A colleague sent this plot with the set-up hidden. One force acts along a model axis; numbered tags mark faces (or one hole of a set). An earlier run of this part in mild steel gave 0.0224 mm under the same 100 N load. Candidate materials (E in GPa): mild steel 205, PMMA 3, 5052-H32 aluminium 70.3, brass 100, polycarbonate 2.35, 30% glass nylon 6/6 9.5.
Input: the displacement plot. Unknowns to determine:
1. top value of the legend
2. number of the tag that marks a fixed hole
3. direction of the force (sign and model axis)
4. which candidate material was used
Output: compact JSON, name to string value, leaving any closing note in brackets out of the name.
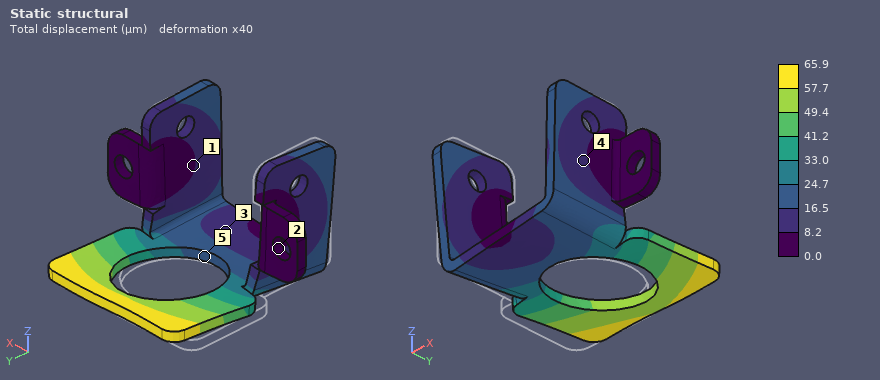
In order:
{"top value of the legend": "65.9 µm", "number of the tag that marks a fixed hole": "2", "direction of the force": "+X", "which candidate material was used": "5052-H32 aluminium"}
